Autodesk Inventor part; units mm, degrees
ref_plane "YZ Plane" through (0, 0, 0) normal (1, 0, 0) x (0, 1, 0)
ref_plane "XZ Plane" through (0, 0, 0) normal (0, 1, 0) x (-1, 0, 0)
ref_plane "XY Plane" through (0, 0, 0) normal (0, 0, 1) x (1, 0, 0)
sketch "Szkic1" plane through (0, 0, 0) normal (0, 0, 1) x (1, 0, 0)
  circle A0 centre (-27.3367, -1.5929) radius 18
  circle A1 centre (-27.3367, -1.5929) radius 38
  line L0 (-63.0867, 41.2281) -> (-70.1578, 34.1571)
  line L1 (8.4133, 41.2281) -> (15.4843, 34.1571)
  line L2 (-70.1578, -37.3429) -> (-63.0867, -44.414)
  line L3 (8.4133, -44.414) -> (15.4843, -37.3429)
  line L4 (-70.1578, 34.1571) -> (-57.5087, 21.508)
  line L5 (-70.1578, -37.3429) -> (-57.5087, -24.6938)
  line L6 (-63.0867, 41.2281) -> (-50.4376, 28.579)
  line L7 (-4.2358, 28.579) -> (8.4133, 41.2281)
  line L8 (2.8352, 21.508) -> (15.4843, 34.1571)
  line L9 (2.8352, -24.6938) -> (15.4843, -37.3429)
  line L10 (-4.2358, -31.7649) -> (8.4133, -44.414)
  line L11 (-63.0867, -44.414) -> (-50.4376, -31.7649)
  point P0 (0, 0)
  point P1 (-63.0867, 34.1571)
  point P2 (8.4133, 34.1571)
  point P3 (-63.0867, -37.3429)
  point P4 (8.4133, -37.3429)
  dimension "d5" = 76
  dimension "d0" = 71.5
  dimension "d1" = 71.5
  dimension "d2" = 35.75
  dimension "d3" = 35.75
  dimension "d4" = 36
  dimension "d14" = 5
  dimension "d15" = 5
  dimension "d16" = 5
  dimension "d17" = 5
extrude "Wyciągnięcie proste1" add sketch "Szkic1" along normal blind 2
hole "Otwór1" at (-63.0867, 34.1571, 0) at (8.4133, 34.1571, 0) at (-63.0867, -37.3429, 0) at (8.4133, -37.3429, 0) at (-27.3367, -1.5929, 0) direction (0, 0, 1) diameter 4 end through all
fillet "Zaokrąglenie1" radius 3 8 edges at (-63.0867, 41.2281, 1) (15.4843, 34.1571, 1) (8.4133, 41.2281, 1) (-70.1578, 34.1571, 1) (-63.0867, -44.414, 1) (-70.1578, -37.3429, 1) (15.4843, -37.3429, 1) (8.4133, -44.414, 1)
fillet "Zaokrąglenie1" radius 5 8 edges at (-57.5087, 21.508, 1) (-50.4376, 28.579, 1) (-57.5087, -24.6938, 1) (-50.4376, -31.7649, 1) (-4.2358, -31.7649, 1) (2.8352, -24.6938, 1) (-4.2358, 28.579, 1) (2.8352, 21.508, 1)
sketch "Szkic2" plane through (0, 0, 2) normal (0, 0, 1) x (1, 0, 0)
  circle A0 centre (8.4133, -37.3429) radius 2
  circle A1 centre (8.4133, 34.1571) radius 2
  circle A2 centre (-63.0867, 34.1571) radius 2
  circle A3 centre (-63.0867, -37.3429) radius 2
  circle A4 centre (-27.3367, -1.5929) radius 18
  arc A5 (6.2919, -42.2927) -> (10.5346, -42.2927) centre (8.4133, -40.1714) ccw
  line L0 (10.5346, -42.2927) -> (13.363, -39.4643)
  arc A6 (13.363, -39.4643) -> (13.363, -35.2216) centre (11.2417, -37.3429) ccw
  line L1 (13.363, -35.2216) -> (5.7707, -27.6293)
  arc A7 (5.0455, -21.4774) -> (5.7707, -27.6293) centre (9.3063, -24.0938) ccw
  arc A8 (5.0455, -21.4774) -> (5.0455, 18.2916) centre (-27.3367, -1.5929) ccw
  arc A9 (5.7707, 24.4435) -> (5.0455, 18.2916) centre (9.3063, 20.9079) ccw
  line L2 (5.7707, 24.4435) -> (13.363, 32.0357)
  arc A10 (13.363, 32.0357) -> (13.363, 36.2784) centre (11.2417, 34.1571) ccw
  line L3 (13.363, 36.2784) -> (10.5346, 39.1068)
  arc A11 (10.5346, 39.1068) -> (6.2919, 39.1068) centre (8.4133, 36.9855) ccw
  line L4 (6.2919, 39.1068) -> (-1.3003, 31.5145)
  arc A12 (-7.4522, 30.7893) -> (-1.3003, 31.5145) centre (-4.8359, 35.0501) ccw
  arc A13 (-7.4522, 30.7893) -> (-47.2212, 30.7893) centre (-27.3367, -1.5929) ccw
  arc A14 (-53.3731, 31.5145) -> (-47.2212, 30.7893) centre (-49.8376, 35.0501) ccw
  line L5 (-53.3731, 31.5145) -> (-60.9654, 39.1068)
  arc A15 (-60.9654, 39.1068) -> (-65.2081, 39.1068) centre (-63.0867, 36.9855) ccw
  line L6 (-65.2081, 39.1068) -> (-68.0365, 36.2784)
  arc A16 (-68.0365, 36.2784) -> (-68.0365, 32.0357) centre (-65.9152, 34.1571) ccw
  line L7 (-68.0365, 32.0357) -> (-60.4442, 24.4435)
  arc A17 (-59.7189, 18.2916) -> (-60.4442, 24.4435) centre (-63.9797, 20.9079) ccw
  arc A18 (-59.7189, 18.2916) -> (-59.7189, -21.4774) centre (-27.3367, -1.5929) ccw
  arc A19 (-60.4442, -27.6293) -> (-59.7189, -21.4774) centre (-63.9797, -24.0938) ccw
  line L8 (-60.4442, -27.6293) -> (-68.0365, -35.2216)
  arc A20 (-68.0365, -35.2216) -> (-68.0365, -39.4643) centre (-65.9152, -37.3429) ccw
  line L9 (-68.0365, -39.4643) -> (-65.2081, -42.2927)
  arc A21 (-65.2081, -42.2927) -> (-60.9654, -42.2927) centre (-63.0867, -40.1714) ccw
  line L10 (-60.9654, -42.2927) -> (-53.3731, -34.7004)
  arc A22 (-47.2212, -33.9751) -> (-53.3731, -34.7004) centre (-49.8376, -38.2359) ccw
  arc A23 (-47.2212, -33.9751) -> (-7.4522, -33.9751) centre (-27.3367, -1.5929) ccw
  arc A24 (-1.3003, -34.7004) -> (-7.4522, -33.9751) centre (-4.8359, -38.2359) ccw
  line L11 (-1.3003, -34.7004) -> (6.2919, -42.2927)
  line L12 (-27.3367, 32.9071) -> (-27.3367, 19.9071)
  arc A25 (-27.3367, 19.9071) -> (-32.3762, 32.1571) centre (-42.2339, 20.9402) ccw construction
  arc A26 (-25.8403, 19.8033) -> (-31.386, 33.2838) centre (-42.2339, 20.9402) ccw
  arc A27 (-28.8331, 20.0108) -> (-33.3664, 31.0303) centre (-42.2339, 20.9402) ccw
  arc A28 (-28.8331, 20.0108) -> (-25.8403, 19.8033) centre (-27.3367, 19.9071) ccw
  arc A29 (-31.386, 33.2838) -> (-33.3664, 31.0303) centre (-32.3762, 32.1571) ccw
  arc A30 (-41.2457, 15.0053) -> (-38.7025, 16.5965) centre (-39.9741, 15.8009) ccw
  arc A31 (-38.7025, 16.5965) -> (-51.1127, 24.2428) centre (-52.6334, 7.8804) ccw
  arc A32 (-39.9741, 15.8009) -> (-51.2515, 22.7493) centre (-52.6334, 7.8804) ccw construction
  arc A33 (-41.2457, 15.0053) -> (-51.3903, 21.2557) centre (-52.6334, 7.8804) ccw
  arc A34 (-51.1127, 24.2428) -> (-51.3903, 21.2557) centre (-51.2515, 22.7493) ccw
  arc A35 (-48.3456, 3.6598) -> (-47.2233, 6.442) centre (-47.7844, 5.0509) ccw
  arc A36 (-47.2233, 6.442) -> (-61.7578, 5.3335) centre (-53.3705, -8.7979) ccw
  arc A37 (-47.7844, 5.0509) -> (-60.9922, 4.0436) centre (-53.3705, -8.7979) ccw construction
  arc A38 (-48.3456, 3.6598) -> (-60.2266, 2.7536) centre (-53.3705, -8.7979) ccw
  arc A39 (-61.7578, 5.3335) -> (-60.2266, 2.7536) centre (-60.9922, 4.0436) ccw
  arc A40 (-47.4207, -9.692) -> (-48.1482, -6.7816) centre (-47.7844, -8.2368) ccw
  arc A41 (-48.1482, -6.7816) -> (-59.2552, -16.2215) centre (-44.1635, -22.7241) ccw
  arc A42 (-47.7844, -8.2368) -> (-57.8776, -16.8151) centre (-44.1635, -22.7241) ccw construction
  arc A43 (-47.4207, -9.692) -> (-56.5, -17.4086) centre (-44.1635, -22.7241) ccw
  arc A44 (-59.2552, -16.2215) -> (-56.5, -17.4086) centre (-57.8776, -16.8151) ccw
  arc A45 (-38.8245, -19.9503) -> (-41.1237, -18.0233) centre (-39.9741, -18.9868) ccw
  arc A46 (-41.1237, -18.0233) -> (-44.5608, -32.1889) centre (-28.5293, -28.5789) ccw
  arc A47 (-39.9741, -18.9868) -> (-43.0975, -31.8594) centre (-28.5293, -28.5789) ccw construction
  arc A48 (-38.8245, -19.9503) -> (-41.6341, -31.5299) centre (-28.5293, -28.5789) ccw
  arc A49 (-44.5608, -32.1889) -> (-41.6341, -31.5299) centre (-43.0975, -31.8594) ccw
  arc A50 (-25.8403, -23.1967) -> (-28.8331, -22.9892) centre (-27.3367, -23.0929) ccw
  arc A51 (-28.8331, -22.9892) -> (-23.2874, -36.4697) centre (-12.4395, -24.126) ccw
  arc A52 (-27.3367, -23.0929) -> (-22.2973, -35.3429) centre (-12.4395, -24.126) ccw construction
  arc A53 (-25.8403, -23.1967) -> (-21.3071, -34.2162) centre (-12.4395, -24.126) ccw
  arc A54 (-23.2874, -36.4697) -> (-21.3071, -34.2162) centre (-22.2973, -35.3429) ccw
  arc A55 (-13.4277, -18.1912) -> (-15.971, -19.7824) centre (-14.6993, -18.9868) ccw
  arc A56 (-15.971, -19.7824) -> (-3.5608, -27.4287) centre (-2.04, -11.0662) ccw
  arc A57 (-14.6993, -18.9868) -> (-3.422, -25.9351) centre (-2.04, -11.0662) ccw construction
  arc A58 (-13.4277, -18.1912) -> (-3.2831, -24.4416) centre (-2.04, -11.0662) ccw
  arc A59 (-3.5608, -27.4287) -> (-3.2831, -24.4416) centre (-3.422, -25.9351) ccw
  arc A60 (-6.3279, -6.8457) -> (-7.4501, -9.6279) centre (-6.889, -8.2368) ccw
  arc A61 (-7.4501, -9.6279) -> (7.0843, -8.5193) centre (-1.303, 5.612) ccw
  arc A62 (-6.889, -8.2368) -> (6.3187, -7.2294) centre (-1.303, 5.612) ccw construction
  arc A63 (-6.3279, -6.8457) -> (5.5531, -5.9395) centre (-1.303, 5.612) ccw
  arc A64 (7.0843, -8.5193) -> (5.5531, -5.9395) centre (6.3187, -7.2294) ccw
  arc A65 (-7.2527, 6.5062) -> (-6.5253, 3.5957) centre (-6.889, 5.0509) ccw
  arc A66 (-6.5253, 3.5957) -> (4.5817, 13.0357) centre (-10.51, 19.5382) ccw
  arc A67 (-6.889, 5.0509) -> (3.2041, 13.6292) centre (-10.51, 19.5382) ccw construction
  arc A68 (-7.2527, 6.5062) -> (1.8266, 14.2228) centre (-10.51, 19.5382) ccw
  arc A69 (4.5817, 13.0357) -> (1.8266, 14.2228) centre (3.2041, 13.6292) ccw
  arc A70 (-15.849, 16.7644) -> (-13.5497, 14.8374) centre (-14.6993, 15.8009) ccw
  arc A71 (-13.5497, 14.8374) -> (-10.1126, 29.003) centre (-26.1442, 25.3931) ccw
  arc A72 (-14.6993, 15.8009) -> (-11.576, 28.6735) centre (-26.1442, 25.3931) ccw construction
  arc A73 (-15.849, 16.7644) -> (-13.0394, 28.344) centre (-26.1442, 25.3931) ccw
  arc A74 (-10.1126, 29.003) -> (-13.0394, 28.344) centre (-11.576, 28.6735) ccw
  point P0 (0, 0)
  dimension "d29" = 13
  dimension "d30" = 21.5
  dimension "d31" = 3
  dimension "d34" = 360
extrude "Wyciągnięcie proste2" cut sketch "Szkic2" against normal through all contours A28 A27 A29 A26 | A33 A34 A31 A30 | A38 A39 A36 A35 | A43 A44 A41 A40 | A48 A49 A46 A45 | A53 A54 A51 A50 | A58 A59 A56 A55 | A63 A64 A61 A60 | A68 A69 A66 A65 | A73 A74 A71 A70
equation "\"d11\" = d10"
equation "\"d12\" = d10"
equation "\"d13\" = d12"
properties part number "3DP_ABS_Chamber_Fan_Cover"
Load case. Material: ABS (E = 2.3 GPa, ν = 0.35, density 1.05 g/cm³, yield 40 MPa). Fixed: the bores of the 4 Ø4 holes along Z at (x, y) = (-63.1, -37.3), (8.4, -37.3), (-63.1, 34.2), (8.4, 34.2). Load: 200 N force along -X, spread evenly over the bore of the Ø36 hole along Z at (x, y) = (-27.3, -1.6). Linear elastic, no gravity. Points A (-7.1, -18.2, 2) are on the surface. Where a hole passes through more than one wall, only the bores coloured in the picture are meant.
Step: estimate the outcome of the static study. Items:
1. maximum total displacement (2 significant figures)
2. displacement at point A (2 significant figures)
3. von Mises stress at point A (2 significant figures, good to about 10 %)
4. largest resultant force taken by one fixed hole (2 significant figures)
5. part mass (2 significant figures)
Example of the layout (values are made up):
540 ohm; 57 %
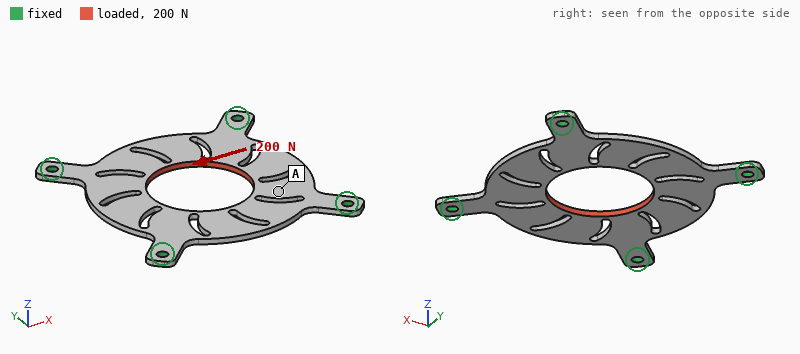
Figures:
0.11 mm; 0.074 mm; 1.7 MPa; 63 N; 7.8 g
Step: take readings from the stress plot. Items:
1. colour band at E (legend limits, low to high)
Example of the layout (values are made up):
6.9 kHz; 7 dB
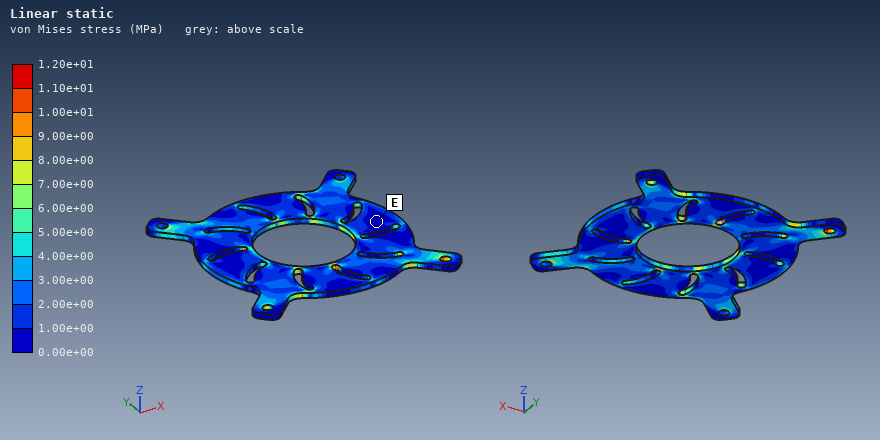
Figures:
0.00e+00 to 1.00e+00 MPa
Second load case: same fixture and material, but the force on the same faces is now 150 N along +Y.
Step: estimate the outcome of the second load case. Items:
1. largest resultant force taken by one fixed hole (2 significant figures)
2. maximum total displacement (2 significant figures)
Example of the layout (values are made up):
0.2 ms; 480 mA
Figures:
44 N; 81 µm
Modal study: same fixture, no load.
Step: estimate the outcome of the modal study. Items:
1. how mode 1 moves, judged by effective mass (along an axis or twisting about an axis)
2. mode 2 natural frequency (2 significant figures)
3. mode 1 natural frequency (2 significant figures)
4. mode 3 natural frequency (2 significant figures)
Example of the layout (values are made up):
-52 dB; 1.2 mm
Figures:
along Z; 550 Hz; 350 Hz; 550 Hz
